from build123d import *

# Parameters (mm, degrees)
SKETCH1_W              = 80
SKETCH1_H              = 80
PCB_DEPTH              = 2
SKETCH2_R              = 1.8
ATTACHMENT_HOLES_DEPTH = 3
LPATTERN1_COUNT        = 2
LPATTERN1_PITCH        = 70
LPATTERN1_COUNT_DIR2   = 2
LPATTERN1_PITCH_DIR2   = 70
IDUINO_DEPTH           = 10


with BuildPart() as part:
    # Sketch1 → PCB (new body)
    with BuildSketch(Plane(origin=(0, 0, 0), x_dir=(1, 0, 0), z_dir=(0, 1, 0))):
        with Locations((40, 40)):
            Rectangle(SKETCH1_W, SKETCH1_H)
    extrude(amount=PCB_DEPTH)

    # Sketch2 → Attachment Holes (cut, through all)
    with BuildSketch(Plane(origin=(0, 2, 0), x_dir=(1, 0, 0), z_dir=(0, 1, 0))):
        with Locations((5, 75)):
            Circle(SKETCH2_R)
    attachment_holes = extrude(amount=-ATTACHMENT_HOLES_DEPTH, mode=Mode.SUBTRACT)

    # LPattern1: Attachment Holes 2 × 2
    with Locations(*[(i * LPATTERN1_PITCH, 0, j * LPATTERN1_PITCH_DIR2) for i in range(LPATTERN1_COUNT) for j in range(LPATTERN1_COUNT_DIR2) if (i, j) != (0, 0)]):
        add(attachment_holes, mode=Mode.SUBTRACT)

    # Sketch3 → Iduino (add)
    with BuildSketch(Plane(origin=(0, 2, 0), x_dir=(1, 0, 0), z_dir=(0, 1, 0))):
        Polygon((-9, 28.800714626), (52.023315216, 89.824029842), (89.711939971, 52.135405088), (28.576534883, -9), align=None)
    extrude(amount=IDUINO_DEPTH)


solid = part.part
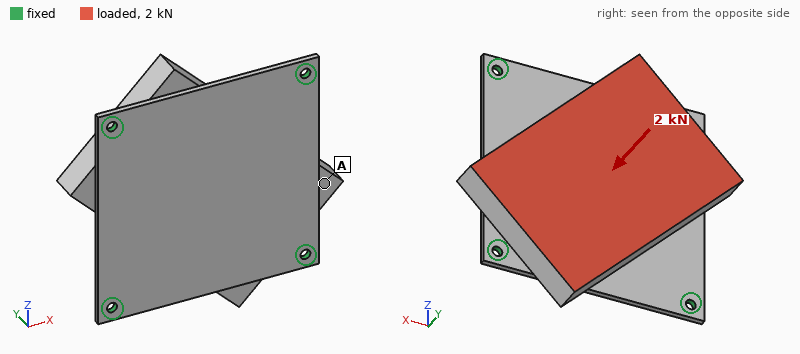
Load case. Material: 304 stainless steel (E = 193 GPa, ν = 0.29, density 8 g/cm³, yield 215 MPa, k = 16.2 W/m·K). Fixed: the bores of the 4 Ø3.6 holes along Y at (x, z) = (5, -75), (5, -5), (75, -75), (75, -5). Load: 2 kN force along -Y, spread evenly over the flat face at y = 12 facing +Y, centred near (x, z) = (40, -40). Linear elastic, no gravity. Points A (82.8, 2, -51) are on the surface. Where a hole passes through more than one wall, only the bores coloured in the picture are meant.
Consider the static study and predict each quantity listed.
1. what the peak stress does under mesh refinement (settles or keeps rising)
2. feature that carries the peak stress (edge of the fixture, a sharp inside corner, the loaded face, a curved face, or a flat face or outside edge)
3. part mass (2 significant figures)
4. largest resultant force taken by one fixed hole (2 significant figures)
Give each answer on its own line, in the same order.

keeps rising
edge of the fixture
470 g
1.3 kN
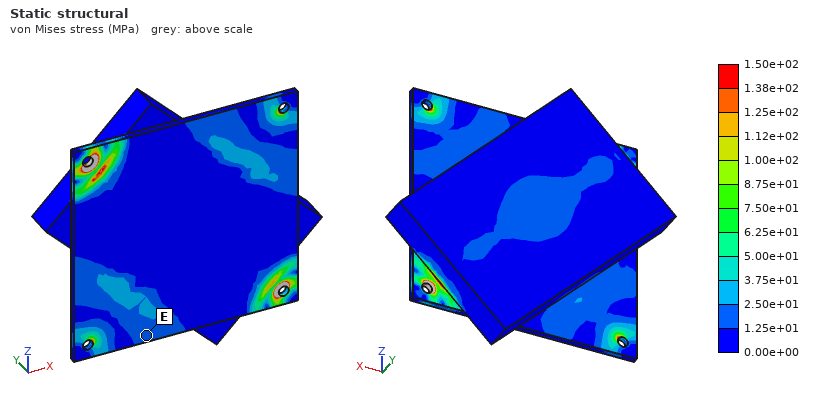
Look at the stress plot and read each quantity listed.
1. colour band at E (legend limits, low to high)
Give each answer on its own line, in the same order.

1.25e+01 to 2.50e+01 MPa
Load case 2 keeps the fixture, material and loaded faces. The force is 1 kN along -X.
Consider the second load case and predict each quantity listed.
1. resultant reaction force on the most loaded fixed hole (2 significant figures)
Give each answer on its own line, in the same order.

330 N
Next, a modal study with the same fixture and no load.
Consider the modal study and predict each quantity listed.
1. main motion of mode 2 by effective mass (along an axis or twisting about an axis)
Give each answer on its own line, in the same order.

along Y
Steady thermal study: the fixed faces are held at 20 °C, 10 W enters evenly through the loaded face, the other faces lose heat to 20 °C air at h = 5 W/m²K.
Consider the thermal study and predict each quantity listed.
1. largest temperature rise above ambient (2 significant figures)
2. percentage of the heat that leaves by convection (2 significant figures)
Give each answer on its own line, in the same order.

46 K
23 %
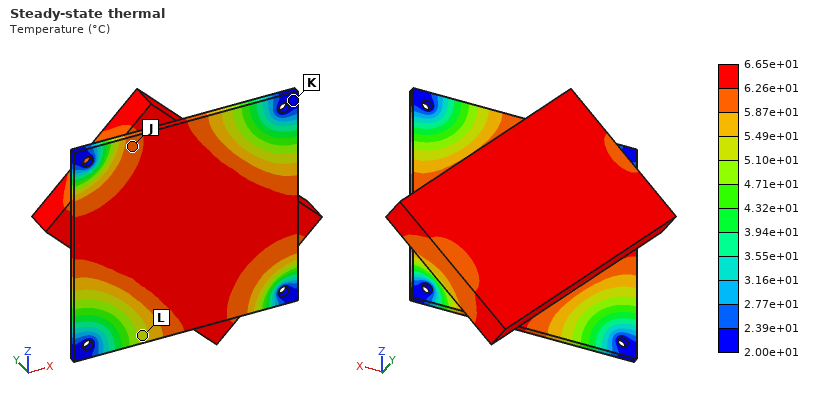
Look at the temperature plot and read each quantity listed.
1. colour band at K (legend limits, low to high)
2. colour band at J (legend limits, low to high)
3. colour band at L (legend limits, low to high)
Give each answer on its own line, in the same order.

2.00e+01 to 2.39e+01 °C
5.87e+01 to 6.26e+01 °C
5.10e+01 to 5.49e+01 °C
